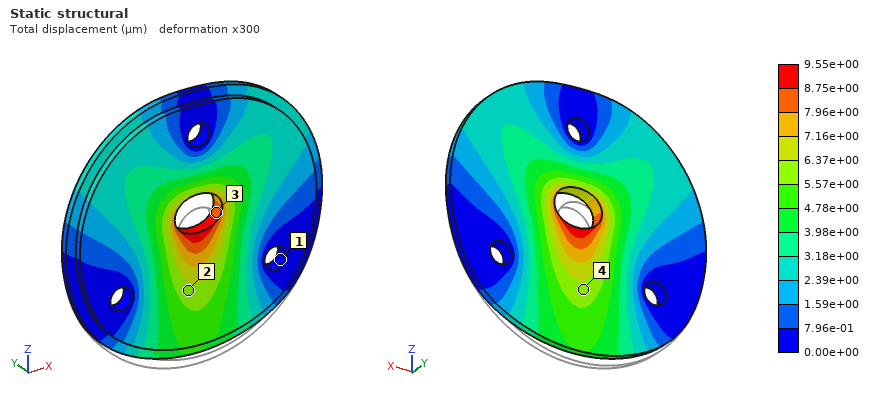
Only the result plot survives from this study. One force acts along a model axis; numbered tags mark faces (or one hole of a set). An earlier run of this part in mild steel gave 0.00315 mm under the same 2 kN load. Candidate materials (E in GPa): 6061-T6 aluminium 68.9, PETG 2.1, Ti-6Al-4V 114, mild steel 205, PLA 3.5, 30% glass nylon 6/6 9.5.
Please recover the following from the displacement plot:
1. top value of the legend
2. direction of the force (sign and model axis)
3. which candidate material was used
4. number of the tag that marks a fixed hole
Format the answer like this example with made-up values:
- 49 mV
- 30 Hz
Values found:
- 9.55e+00 µm
- +Z
- 6061-T6 aluminium
- 1
